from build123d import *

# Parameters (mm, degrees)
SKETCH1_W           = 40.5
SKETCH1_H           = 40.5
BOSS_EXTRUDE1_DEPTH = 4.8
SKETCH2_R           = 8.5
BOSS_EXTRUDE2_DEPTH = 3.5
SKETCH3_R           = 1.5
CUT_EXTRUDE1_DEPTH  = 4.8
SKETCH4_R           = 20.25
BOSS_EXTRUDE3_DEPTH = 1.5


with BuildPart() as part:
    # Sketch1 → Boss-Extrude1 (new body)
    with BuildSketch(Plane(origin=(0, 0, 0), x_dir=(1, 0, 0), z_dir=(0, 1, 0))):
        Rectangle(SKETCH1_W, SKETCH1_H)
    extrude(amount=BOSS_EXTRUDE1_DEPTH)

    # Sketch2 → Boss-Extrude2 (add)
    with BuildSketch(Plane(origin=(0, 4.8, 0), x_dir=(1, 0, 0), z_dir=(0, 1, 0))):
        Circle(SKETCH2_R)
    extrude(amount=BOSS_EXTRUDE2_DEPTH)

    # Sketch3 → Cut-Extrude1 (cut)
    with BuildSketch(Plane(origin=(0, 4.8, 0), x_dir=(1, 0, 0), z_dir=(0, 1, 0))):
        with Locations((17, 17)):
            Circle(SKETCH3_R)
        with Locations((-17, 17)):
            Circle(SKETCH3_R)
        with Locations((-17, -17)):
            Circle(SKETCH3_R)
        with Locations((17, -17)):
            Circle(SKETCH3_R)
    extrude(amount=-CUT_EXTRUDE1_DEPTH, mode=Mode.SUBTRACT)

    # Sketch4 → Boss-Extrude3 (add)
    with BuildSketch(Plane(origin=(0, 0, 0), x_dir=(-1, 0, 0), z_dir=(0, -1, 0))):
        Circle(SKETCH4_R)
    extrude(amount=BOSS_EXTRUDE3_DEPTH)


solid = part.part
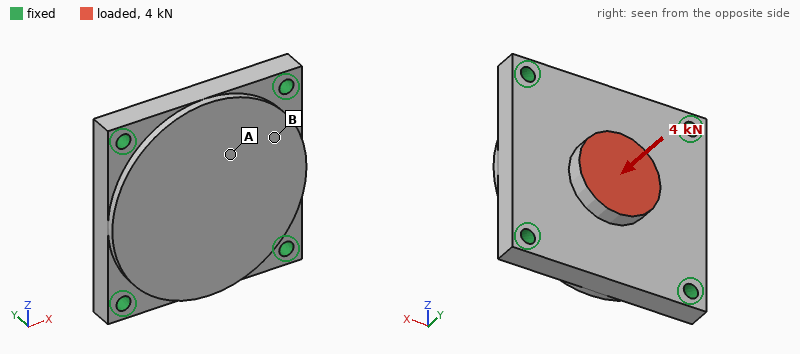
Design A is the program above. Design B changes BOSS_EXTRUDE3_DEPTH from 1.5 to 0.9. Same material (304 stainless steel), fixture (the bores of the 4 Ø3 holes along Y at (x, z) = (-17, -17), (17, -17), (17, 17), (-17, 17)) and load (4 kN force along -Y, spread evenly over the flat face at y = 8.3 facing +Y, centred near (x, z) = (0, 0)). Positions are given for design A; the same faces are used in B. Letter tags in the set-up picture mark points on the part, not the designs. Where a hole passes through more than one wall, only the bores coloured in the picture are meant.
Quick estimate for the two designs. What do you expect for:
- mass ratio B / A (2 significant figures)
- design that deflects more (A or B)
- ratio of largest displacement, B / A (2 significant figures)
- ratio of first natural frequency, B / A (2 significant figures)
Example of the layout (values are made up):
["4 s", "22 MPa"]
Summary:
["0.93", "B", "1.2", "0.97"]
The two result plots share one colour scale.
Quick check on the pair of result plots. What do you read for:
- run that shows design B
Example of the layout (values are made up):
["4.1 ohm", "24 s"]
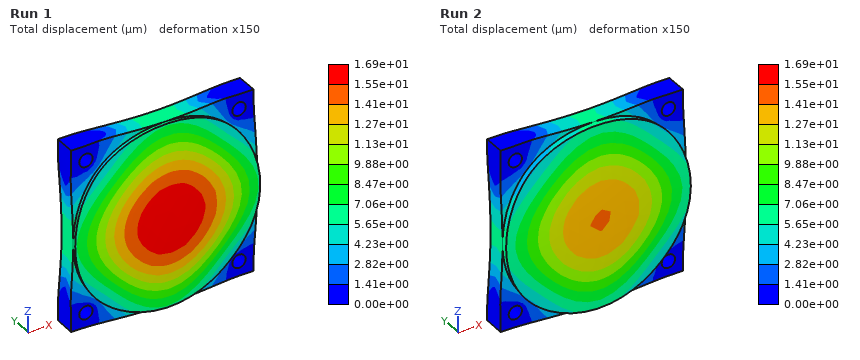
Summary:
["Run 1"]
